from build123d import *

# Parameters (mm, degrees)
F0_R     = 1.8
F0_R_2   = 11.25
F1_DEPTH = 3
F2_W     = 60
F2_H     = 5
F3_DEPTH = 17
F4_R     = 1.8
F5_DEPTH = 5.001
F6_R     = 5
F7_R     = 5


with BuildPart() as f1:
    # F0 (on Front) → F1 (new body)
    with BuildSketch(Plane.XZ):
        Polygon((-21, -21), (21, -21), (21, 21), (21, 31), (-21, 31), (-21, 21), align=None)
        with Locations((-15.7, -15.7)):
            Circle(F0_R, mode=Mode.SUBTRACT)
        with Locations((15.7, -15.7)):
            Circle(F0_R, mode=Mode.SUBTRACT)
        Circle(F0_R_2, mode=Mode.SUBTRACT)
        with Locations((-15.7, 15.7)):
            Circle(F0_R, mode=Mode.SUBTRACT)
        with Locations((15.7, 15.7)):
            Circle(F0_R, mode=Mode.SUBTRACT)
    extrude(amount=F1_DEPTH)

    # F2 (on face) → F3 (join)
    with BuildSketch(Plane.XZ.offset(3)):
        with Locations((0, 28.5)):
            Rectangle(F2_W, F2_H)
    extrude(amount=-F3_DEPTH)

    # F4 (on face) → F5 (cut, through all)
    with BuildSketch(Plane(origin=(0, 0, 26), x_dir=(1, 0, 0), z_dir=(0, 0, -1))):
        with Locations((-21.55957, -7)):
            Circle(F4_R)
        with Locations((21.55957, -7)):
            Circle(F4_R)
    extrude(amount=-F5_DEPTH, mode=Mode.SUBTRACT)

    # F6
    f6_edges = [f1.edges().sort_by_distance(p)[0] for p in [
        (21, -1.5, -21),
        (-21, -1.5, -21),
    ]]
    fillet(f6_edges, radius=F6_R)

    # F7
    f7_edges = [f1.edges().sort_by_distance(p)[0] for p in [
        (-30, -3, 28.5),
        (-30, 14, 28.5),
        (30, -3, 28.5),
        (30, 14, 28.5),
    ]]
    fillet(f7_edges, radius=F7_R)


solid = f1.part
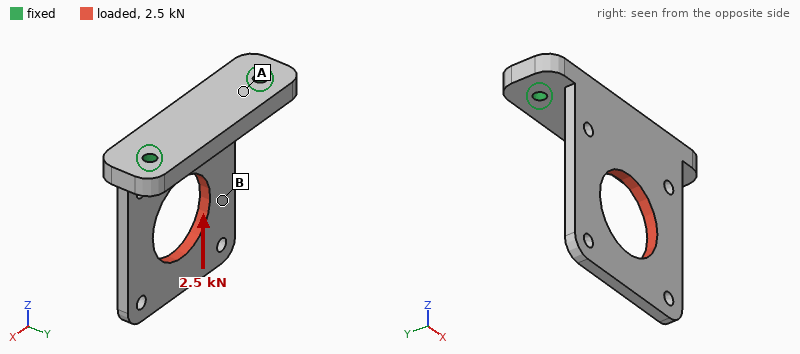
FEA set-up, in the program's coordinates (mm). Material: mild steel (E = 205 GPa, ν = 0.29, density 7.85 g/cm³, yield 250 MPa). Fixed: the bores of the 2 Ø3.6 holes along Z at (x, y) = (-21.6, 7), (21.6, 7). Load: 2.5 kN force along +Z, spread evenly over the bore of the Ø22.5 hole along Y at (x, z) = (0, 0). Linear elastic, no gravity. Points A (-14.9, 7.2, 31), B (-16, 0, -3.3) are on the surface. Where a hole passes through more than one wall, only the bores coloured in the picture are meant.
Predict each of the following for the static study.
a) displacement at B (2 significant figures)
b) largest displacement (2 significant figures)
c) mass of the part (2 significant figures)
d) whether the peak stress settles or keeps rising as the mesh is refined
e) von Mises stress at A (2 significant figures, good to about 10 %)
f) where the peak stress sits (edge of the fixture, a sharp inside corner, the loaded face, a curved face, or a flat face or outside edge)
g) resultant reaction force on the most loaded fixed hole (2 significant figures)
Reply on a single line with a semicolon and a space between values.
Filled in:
49 µm; 76 µm; 74 g; keeps rising; 46 MPa; edge of the fixture; 1.3 kN
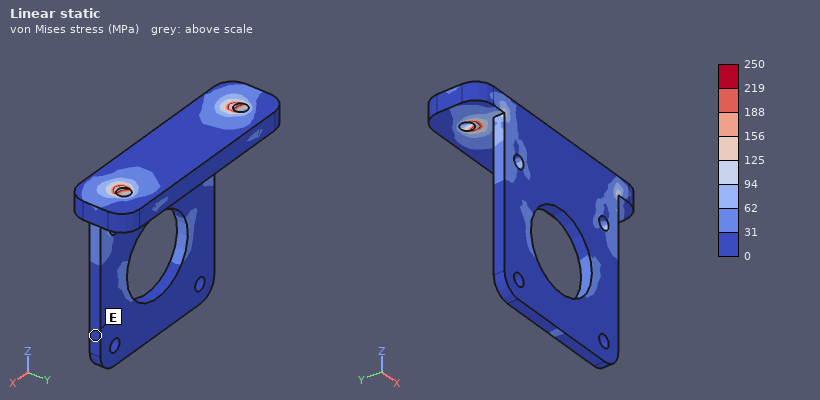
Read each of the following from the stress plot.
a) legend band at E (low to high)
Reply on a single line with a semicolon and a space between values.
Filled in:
0 to 31 MPa
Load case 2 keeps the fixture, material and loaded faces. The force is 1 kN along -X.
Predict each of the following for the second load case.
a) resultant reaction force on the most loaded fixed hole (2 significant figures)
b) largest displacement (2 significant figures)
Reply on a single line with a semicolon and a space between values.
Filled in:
880 N; 31 µm
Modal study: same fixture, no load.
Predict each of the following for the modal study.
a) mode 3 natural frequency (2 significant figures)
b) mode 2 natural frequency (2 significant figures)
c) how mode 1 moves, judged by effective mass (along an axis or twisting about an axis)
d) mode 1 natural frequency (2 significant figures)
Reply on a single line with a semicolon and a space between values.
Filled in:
5500 Hz; 2500 Hz; along Y; 990 Hz
